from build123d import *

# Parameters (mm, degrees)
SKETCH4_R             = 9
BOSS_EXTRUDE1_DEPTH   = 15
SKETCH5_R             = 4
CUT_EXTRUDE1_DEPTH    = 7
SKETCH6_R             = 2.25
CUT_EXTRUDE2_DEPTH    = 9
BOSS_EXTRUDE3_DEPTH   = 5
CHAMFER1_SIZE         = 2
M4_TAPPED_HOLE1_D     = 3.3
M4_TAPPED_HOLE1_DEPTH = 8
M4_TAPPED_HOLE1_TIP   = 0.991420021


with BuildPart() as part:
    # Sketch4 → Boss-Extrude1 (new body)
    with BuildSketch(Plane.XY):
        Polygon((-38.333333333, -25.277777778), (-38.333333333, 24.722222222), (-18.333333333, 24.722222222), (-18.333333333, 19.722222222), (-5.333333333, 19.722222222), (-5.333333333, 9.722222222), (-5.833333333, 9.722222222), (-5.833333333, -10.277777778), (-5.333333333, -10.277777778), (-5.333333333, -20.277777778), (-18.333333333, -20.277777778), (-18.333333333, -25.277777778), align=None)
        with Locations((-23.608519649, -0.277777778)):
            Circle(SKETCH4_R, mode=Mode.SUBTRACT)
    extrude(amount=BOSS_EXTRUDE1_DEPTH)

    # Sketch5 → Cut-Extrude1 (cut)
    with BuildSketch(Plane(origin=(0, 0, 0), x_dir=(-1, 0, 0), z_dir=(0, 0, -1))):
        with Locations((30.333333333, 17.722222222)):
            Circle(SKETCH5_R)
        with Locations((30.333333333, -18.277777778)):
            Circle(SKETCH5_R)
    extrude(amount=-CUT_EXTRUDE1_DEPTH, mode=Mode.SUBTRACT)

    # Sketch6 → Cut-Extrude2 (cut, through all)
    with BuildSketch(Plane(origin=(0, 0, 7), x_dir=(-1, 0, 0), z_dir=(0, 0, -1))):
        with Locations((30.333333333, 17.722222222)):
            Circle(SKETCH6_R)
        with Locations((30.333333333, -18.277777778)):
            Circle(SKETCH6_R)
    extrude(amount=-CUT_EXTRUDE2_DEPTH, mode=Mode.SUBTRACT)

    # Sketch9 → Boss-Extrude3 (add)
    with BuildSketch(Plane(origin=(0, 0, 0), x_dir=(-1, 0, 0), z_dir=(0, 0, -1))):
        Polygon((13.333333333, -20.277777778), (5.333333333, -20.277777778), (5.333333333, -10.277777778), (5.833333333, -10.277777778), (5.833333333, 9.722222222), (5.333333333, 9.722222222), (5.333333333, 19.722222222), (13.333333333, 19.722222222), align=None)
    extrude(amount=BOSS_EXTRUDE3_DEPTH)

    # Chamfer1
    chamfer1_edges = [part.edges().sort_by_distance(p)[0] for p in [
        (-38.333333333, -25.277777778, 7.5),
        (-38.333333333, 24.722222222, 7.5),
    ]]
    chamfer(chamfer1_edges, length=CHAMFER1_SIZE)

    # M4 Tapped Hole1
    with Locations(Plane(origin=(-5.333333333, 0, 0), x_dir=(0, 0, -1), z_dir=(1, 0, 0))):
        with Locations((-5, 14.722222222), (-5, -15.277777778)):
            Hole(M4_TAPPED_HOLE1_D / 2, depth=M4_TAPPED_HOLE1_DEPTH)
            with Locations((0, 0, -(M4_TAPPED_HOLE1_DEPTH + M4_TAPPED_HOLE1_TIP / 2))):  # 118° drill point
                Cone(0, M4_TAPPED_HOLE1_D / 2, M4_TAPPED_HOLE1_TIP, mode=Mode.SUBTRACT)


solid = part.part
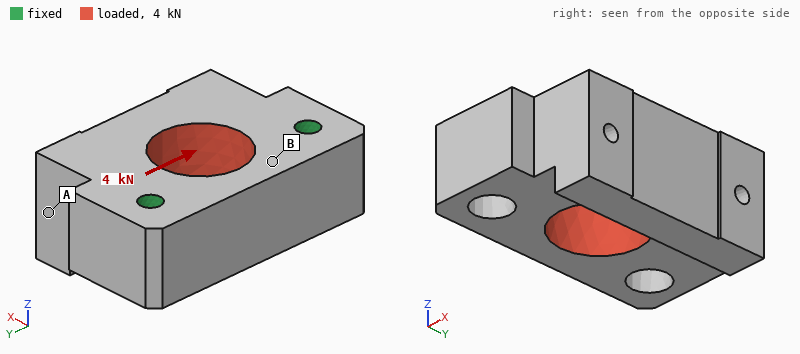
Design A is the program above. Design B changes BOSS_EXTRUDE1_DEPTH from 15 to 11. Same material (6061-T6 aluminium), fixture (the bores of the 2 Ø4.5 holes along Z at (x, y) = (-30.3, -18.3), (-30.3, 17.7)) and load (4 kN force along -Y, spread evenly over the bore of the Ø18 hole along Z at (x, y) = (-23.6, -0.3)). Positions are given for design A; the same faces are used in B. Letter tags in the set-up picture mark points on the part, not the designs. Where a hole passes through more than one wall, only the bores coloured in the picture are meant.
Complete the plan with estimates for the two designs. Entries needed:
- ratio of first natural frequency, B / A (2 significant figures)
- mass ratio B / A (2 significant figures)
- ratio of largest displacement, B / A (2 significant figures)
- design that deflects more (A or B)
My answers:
0.64
0.75
1.6
B
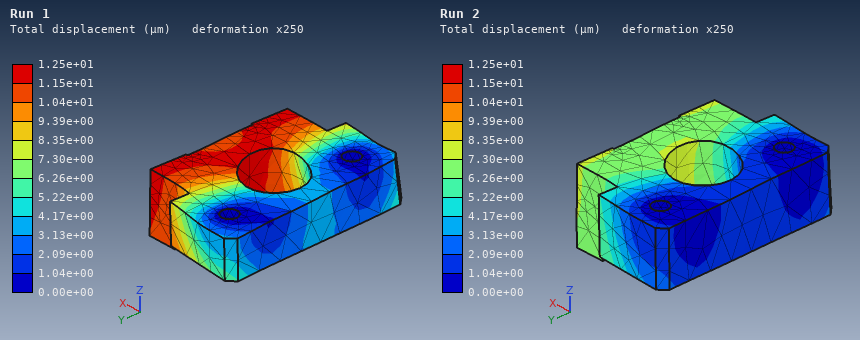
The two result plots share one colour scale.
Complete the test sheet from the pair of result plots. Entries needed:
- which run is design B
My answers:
Run 1
